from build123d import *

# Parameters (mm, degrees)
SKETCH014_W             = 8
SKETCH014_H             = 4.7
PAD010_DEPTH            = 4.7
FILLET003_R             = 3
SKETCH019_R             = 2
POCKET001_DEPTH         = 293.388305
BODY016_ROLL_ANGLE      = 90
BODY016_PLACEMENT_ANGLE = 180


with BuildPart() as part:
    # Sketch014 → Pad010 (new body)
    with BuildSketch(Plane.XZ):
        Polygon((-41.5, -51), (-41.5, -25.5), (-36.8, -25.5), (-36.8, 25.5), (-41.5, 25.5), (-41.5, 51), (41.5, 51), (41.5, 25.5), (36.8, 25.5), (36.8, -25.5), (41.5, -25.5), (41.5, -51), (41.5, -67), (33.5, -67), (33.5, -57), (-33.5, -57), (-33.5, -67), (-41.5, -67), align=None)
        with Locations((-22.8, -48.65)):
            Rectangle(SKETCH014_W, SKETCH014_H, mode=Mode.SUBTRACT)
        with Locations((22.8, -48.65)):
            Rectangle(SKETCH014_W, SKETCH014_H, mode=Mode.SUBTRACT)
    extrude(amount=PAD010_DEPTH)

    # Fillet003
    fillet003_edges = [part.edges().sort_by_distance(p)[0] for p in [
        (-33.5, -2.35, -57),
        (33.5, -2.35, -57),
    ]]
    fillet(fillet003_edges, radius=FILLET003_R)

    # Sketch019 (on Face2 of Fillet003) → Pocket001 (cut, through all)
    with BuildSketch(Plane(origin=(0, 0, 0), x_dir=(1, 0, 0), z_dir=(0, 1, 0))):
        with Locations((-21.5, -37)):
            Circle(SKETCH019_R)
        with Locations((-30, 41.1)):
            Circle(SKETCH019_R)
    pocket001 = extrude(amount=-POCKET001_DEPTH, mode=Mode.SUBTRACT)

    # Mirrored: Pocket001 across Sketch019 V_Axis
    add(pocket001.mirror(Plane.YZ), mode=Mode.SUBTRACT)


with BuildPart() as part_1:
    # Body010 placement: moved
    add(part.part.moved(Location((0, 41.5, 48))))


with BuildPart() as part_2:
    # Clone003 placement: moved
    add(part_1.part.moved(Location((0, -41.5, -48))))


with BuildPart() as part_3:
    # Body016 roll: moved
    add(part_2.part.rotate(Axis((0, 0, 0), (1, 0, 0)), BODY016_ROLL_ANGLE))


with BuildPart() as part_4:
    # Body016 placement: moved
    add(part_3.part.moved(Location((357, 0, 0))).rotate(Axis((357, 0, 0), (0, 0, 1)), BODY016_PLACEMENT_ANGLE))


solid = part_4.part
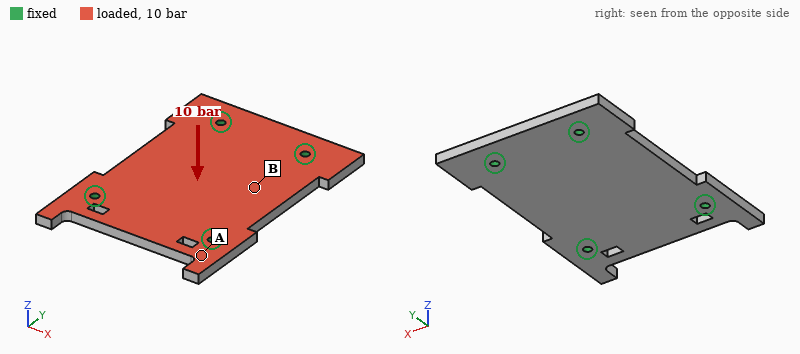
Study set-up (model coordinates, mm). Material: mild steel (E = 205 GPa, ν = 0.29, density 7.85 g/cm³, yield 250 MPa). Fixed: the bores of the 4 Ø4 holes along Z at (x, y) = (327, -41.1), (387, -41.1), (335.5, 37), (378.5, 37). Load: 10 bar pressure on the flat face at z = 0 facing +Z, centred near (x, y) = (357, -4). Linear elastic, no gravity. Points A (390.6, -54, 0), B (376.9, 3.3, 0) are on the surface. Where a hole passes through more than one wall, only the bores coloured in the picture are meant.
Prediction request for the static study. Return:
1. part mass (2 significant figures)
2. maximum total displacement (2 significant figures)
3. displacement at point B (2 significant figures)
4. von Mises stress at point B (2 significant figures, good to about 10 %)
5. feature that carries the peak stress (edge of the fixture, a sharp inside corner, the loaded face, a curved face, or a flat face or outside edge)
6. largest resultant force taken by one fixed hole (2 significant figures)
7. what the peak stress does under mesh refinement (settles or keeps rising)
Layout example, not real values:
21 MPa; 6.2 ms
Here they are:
310 g; 80 µm; 70 µm; 66 MPa; edge of the fixture; 2.2 kN; keeps rising
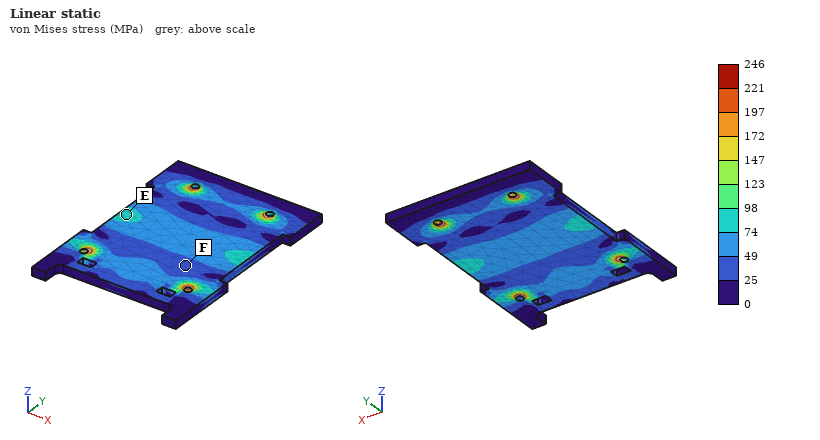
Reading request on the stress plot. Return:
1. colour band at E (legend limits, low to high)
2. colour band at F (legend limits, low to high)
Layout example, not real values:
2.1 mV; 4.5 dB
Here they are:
74 to 98 MPa; 25 to 49 MPa
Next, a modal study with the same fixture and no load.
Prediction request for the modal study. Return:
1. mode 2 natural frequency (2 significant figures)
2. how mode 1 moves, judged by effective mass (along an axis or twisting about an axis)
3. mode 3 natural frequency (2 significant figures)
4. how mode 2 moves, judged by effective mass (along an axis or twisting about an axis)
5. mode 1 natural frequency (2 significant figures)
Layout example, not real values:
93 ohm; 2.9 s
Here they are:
4600 Hz; along Z; 5600 Hz; twisting about Y; 3300 Hz
